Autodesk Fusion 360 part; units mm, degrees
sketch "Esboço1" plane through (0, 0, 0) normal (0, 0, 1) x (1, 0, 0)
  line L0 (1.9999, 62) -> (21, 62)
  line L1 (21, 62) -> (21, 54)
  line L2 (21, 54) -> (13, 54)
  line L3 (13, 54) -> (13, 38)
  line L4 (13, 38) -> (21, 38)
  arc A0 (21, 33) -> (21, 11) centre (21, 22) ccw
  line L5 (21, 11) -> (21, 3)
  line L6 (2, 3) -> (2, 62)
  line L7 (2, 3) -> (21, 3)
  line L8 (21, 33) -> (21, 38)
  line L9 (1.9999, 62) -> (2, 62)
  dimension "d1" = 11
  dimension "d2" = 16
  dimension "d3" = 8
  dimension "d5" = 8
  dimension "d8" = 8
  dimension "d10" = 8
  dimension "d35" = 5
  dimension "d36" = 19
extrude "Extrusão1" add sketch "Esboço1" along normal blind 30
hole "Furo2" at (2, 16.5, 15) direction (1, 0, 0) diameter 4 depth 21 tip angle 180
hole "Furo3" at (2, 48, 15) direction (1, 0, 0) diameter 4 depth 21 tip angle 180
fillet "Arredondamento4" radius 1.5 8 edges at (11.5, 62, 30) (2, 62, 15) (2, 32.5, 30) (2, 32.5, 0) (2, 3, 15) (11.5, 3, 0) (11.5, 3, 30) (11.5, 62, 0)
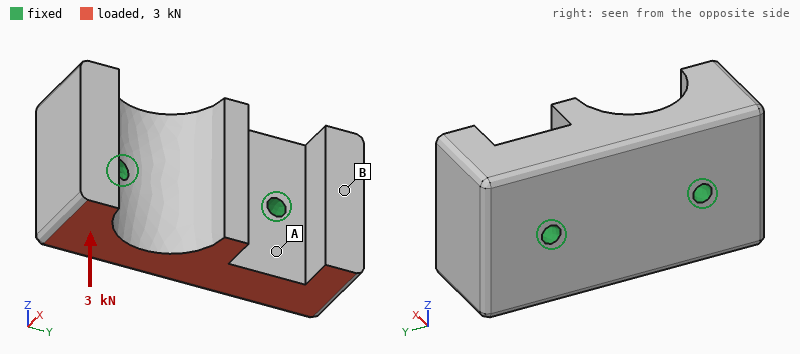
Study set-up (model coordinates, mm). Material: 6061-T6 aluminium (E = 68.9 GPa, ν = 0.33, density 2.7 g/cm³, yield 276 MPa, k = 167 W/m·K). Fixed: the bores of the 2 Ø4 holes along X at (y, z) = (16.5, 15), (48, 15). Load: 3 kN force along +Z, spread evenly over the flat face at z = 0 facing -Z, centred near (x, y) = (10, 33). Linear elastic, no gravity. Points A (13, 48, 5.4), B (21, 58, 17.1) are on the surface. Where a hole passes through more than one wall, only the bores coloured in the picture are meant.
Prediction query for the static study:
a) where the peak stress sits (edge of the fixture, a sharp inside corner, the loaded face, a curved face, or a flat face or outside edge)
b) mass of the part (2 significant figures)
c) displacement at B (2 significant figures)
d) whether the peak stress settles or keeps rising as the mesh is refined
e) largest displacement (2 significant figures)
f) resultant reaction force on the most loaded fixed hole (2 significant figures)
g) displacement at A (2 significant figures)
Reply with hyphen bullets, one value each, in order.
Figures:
- edge of the fixture
- 64 g
- 3.7 µm
- keeps rising
- 5.8 µm
- 1.6 kN
- 2.5 µm
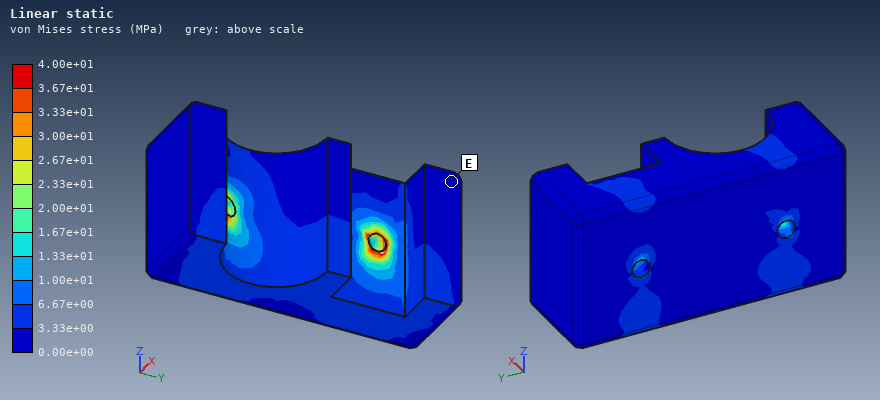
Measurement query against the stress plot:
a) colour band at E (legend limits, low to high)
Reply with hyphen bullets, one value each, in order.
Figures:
- 0.00e+00 to 3.33e+00 MPa
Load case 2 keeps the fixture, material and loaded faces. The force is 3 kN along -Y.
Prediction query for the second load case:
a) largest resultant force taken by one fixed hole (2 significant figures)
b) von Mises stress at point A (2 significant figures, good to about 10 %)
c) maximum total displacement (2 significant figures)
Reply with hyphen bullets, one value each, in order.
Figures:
- 2.0 kN
- 12 MPa
- 12 µm
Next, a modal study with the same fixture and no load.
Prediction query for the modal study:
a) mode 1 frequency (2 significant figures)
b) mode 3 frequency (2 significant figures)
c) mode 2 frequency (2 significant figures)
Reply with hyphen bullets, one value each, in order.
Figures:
- 14 kHz
- 17 kHz
- 17 kHz
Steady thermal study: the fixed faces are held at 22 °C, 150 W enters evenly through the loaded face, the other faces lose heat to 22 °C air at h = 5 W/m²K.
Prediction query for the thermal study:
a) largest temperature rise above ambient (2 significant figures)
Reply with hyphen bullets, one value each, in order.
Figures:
- 29 K
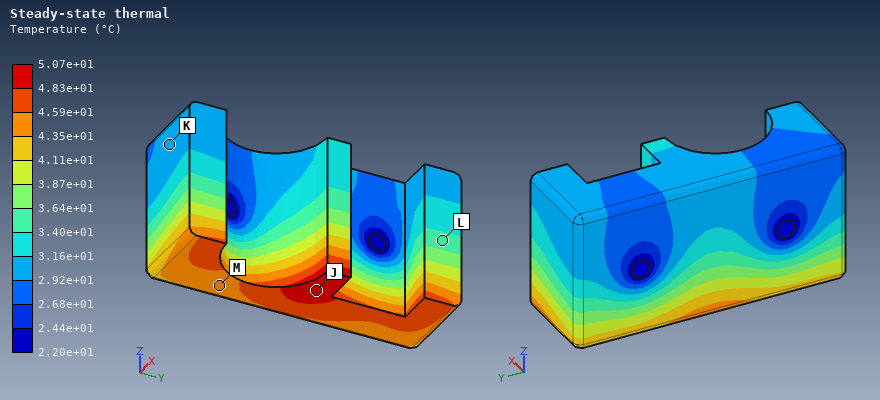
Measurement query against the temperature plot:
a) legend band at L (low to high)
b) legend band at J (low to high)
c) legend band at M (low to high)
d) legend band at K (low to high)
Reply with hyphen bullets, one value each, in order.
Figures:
- 3.40e+01 to 3.64e+01 °C
- 4.83e+01 to 5.07e+01 °C
- 4.35e+01 to 4.59e+01 °C
- 2.92e+01 to 3.16e+01 °C
